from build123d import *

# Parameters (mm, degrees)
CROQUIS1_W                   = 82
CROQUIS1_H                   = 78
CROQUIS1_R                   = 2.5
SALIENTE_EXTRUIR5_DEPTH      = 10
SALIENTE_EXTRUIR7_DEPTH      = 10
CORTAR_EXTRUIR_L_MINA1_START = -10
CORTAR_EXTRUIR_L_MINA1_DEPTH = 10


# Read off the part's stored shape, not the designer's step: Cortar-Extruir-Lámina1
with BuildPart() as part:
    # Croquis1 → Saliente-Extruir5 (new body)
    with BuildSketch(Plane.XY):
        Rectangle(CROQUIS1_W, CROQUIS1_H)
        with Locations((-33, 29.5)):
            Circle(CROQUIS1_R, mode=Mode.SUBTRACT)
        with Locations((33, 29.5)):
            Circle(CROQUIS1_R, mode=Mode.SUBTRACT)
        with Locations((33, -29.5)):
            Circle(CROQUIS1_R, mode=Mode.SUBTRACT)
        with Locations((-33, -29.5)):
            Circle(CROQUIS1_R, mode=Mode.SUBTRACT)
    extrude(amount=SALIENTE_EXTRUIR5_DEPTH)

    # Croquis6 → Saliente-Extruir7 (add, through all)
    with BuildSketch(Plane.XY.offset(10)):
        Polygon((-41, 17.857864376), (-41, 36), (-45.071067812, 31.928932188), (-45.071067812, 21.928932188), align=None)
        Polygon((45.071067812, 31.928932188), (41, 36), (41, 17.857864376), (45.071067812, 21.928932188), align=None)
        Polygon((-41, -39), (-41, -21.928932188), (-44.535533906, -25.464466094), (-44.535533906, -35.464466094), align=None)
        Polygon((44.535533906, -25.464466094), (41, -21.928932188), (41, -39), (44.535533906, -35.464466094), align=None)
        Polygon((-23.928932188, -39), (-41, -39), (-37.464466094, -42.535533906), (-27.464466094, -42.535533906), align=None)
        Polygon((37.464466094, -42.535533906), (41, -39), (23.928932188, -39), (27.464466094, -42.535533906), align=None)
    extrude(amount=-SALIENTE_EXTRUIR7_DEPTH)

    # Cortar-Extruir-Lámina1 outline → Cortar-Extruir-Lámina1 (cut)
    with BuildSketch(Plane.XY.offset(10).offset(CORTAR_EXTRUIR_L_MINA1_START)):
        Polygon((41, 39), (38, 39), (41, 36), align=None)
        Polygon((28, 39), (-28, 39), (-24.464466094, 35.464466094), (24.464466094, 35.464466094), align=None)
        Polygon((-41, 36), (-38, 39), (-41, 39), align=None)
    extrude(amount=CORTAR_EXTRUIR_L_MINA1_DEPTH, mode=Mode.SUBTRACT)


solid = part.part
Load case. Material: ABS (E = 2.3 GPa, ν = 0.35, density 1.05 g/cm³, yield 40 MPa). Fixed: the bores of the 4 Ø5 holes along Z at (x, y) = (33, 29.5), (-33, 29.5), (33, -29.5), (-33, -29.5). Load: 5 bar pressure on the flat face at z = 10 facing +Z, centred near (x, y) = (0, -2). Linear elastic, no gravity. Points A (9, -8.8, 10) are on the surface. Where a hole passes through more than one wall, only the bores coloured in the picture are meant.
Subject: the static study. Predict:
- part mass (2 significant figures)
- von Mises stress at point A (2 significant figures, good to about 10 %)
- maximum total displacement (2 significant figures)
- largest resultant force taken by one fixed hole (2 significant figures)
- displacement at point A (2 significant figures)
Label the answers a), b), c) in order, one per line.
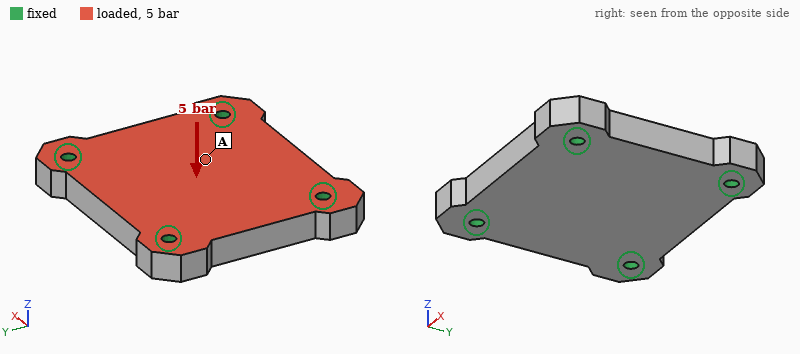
a) 68 g
b) 5.4 MPa
c) 0.32 mm
d) 840 N
e) 0.30 mm
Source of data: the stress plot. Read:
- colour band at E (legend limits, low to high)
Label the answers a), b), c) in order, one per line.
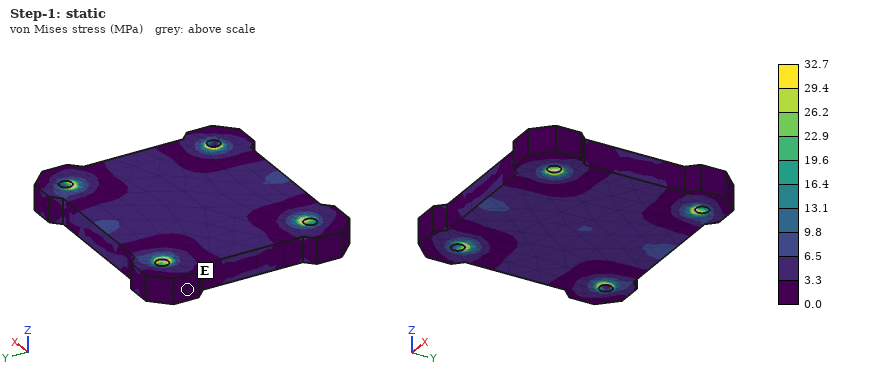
a) 0.0 to 3.3 MPa
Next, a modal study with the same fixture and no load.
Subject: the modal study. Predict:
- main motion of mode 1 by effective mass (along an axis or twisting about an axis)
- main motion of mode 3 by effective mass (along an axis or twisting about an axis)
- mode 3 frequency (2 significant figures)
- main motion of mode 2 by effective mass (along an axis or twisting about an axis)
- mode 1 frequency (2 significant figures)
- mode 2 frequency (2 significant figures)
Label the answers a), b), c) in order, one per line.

a) along Z
b) twisting about Y
c) 3900 Hz
d) twisting about X
e) 2300 Hz
f) 3400 Hz
